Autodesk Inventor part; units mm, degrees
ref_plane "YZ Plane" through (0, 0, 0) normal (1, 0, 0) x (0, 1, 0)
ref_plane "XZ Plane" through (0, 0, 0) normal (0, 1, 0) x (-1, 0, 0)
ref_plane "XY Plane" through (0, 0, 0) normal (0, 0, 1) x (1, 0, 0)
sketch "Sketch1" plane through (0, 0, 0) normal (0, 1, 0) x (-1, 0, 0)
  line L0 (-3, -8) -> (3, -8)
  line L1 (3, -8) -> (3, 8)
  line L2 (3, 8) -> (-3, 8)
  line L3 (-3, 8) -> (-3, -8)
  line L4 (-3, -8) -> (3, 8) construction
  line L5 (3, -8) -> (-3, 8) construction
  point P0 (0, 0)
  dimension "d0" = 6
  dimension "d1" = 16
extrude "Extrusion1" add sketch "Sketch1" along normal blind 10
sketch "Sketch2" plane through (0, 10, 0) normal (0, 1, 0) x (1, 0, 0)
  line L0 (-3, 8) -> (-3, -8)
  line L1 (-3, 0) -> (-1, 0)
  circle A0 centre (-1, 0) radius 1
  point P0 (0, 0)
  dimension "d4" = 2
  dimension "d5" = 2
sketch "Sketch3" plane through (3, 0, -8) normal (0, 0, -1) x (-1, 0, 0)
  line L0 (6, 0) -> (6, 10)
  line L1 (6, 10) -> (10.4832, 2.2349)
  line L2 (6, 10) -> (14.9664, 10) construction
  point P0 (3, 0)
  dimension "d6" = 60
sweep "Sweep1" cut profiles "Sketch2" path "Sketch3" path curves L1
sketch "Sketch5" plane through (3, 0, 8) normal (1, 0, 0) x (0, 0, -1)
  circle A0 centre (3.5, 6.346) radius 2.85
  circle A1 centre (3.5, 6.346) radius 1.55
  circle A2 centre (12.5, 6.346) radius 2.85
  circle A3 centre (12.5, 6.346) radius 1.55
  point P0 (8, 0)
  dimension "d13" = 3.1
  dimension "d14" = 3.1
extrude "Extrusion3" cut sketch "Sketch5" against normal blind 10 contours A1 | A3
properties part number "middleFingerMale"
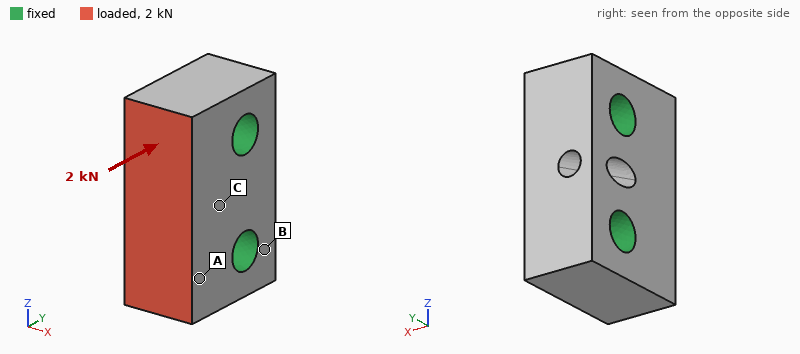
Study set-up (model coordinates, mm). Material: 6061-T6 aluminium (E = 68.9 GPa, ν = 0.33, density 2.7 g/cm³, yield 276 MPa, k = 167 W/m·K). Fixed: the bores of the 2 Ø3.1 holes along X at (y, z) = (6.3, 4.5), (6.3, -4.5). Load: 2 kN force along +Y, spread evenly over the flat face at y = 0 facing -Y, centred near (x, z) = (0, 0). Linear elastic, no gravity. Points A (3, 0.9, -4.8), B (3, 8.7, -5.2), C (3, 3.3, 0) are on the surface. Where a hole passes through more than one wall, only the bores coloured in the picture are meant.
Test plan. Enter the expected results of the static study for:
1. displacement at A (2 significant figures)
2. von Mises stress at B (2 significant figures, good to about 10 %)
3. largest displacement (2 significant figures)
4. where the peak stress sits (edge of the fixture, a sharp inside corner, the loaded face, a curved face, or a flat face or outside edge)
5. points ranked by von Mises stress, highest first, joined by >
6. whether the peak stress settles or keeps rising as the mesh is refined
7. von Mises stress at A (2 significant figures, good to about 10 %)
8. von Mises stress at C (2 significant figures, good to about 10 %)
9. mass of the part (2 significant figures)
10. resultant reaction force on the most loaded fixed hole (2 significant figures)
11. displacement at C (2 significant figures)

1.6 µm
3.8 MPa
2.3 µm
edge of the fixture
A > C > B
keeps rising
22 MPa
12 MPa
2.3 g
1.0 kN
1.1 µm
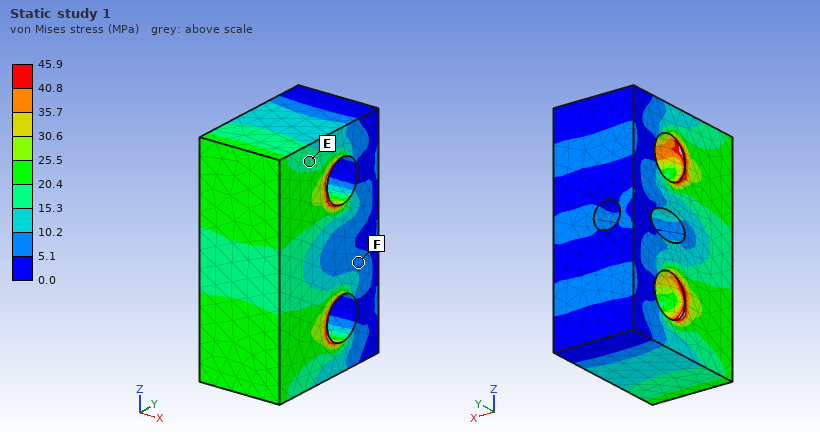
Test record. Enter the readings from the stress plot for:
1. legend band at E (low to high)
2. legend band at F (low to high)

15.3 to 20.4 MPa
5.1 to 10.2 MPa
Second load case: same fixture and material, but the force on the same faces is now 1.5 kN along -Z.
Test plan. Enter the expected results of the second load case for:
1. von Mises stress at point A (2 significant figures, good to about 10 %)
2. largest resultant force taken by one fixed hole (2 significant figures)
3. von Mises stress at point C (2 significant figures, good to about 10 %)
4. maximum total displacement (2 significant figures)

31 MPa
1.0 kN
39 MPa
7.3 µm
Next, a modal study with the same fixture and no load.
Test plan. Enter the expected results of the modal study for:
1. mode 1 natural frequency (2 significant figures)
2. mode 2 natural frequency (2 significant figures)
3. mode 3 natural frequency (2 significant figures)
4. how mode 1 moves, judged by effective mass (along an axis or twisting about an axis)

91 kHz
110 kHz
110 kHz
along X
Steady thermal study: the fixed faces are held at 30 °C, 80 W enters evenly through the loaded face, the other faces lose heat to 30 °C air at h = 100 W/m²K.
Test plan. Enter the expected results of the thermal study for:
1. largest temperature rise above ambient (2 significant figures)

29 K
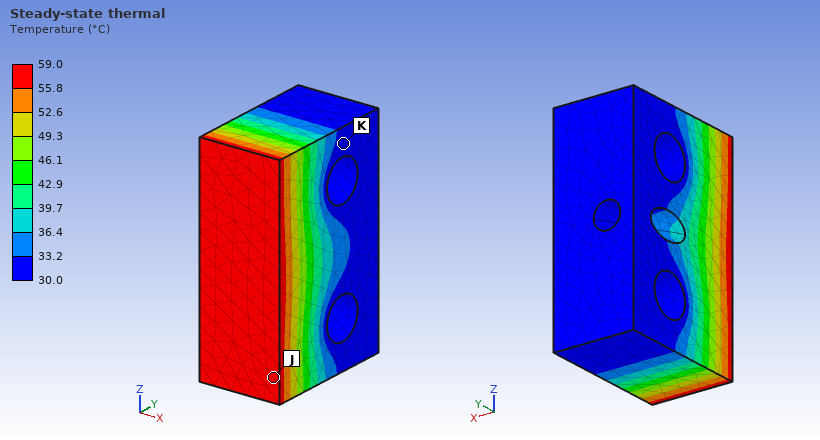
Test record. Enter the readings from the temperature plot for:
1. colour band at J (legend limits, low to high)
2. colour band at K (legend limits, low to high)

55.8 to 59.0 °C
30.0 to 33.2 °C
